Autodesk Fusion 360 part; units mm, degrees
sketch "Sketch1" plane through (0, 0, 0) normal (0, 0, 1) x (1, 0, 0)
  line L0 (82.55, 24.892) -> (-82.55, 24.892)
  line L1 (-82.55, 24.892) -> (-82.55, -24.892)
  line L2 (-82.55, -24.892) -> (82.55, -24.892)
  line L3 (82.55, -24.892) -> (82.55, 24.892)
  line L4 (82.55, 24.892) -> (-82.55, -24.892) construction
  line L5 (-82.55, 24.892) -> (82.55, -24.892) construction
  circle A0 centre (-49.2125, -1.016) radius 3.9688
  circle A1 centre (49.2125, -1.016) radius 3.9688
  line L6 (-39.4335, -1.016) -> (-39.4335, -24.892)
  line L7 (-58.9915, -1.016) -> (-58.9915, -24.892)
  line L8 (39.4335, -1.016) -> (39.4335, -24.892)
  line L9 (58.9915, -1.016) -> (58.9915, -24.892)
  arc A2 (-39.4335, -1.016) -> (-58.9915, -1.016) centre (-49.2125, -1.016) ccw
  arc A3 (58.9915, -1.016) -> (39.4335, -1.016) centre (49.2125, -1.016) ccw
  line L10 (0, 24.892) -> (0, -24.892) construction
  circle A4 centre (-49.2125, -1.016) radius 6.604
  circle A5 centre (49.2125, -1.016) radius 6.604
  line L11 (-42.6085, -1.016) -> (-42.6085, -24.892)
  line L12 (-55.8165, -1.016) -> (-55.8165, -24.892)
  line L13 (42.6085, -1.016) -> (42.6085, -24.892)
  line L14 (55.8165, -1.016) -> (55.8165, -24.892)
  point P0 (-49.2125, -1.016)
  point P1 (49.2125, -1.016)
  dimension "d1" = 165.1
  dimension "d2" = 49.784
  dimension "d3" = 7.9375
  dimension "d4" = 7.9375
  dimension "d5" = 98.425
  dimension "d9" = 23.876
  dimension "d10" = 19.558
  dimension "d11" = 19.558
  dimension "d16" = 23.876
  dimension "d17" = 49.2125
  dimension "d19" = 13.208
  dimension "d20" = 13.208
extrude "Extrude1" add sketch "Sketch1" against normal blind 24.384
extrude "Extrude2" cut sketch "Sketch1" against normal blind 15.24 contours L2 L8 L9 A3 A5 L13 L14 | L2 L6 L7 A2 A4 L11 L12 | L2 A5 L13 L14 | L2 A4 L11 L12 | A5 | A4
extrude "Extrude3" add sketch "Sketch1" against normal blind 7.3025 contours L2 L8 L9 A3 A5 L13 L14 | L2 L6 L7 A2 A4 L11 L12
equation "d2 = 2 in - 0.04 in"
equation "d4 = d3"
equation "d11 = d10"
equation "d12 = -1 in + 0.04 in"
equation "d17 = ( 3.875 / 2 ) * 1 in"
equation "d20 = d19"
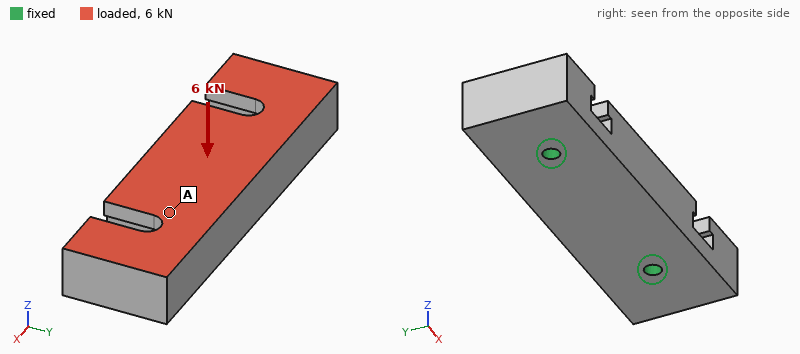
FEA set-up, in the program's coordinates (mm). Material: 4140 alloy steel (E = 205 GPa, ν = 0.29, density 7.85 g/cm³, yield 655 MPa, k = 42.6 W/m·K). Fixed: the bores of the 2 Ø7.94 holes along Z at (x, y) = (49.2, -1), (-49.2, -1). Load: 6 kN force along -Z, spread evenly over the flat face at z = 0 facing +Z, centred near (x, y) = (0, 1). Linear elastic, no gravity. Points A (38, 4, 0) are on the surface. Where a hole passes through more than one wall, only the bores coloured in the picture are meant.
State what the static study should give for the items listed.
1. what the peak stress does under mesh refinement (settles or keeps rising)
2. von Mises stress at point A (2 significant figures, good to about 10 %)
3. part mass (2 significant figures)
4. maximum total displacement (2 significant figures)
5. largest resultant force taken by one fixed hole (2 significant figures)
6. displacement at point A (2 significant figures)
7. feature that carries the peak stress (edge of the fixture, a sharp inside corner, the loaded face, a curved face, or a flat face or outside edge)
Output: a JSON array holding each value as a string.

["keeps rising", "4.4 MPa", "1.4 kg", "3.9 µm", "3.1 kN", "2.1 µm", "edge of the fixture"]
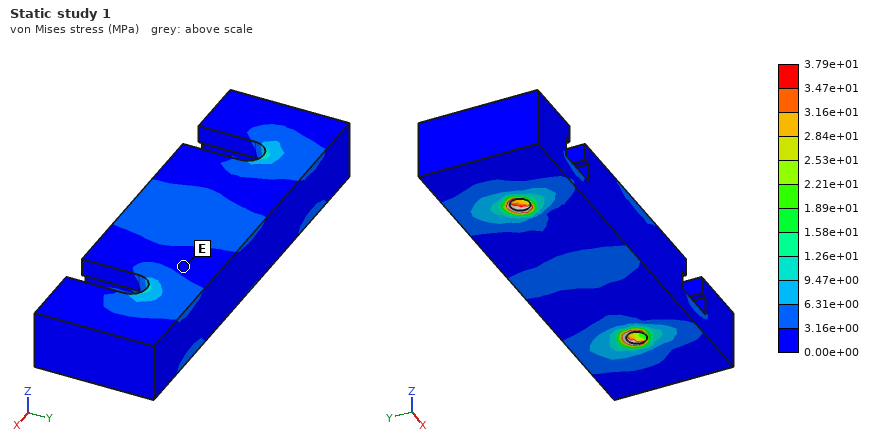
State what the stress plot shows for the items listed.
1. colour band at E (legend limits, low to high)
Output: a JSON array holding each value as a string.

["0.00e+00 to 3.16e+00 MPa"]
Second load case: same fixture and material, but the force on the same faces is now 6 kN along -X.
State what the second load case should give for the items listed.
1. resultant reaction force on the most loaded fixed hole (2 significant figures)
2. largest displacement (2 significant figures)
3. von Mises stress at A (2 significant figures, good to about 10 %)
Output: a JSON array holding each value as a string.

["3.2 kN", "5.7 µm", "5.2 MPa"]
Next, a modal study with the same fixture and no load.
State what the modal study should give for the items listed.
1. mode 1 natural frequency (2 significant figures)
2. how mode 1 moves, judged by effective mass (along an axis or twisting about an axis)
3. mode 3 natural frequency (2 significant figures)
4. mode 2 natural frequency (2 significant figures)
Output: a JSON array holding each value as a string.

["3500 Hz", "along Y", "5700 Hz", "5300 Hz"]
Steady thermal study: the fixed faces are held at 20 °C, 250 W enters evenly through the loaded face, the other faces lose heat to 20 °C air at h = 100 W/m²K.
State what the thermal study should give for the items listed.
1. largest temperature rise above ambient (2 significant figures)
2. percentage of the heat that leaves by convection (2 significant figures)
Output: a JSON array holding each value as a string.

["73 K", "42 %"]
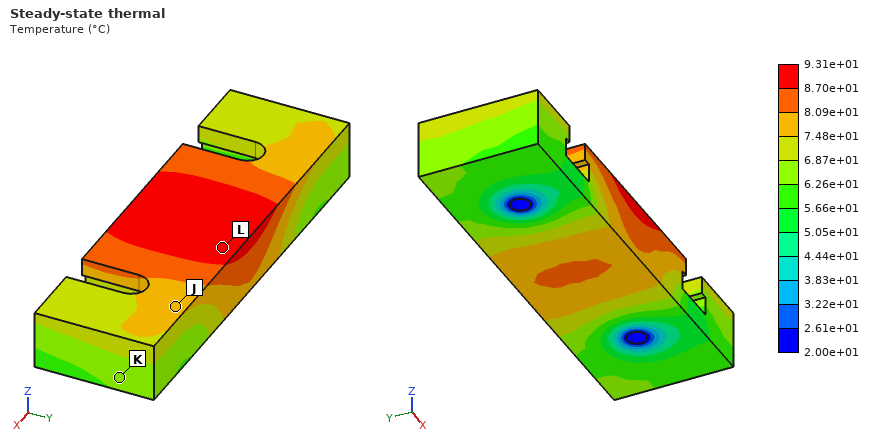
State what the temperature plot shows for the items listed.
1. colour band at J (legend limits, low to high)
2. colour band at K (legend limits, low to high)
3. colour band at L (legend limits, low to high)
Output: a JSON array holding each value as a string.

["7.48e+01 to 8.09e+01 °C", "6.26e+01 to 6.87e+01 °C", "8.70e+01 to 9.31e+01 °C"]
